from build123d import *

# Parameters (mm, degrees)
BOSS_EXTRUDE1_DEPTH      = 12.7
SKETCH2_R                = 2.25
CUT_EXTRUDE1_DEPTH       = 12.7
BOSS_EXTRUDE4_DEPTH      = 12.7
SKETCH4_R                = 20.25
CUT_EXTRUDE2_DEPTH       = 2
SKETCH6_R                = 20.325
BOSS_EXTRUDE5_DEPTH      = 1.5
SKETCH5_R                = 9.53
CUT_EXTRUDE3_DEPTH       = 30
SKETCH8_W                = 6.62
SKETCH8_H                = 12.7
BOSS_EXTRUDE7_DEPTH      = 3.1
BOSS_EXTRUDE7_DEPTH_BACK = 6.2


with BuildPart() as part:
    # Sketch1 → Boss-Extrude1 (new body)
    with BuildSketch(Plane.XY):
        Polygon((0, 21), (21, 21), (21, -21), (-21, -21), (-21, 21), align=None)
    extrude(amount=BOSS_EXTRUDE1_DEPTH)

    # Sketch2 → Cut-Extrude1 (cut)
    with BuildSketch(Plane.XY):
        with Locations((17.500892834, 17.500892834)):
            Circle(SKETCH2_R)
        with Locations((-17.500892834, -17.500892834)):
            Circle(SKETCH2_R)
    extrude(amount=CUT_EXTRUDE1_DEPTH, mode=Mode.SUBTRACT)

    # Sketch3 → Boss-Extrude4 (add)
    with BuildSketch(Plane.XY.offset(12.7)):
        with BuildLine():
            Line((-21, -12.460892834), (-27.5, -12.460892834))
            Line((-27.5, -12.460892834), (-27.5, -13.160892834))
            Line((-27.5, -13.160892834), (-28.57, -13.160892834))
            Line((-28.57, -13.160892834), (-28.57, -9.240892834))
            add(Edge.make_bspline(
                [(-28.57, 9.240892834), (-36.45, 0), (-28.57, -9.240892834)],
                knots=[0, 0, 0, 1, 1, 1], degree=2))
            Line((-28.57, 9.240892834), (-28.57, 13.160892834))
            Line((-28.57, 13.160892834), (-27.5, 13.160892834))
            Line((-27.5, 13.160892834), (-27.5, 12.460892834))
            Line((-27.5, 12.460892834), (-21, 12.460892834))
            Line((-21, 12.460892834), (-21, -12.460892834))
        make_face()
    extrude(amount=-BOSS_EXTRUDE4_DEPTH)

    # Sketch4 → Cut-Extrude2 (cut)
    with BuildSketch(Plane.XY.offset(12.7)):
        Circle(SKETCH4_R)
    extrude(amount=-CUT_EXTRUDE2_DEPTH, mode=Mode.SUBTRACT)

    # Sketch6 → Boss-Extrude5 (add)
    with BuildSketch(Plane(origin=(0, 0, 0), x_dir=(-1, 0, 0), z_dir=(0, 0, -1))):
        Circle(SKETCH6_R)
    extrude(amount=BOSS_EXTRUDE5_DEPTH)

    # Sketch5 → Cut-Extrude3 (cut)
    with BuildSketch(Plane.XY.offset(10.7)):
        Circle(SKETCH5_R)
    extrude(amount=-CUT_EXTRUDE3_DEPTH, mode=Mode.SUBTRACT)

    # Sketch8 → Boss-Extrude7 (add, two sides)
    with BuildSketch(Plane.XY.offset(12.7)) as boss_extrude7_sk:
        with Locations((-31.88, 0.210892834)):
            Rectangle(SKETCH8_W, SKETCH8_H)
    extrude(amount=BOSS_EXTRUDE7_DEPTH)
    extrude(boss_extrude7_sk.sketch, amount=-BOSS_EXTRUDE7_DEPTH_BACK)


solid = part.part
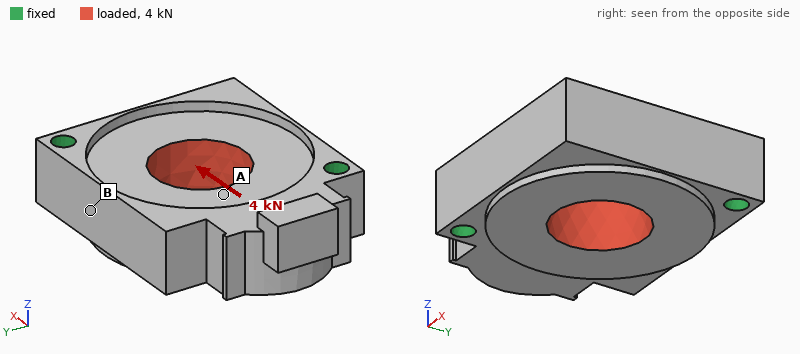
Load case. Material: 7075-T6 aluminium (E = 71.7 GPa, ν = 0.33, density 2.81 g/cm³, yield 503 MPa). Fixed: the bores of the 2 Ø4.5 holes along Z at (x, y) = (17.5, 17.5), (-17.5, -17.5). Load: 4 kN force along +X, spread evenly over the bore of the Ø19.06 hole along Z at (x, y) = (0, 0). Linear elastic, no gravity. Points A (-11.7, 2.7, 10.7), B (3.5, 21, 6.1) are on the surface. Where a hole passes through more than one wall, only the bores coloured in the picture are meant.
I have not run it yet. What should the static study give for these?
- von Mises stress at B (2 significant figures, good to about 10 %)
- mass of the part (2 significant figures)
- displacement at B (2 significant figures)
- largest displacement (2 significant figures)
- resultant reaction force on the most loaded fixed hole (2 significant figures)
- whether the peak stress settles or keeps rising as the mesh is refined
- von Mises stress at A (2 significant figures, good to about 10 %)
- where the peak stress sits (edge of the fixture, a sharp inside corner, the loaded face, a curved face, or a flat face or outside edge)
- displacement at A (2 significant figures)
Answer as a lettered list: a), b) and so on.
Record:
a) 14 MPa
b) 60 g
c) 3.0 µm
d) 6.6 µm
e) 2.0 kN
f) keeps rising
g) 5.4 MPa
h) edge of the fixture
i) 4.2 µm
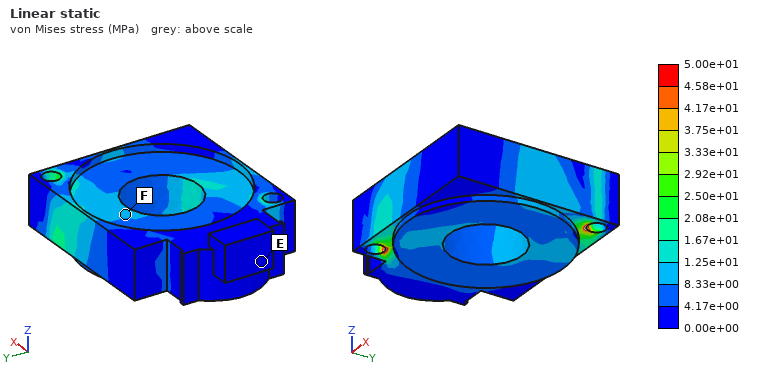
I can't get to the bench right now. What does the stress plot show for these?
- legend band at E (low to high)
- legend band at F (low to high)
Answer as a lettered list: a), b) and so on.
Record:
a) 0.00e+00 to 4.17e+00 MPa
b) 8.33e+00 to 1.25e+01 MPa
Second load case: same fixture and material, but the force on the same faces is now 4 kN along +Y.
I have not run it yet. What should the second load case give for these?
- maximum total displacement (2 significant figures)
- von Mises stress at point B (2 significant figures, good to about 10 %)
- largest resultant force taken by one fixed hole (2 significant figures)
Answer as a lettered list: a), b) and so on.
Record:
a) 6.6 µm
b) 12 MPa
c) 2.0 kN
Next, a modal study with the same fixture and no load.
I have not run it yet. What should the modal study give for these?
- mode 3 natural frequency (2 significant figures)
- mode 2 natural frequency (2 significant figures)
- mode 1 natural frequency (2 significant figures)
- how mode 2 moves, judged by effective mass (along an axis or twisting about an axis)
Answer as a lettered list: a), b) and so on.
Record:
a) 17 kHz
b) 10 kHz
c) 7500 Hz
d) along Z
